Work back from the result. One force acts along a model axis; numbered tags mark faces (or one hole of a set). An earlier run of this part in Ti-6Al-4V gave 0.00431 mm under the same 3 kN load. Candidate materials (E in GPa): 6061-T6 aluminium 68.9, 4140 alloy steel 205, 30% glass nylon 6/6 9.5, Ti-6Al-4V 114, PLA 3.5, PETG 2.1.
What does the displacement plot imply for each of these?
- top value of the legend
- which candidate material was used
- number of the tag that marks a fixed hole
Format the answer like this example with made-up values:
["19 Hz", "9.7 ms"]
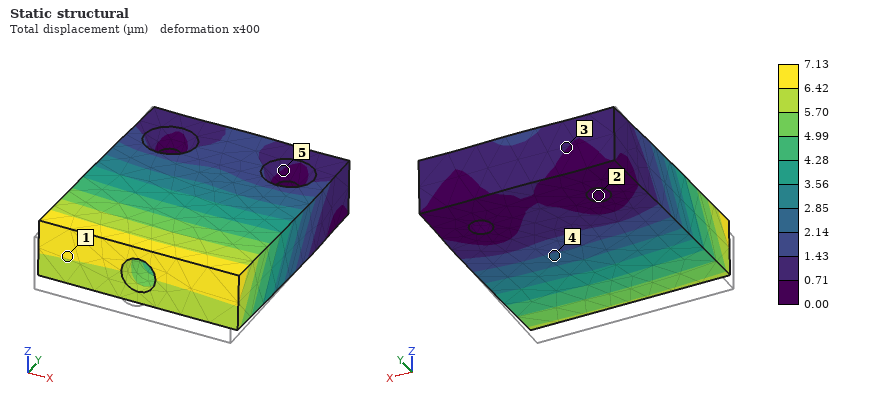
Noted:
["7.13 µm", "6061-T6 aluminium", "2"]
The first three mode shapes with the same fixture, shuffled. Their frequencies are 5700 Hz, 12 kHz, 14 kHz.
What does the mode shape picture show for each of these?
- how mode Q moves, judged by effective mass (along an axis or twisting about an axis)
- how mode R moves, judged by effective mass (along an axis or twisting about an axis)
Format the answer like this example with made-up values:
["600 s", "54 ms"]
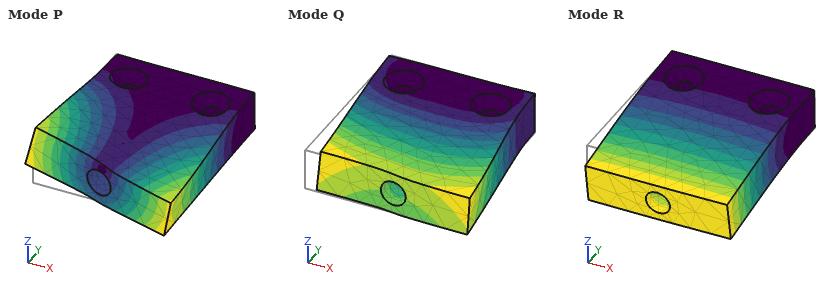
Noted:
["along X", "along Z"]
